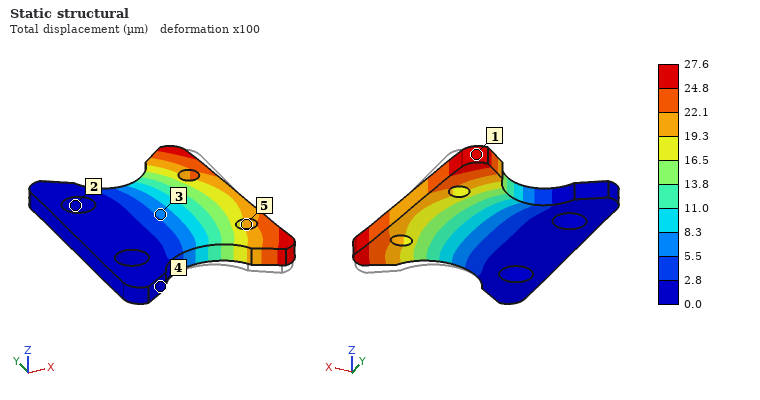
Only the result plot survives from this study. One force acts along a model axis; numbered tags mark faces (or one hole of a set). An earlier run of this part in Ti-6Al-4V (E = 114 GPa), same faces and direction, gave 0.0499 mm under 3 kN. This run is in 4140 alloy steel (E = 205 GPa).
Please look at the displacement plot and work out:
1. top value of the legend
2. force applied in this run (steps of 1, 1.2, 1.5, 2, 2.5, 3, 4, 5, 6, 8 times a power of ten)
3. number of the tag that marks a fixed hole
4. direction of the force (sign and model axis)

27.6 µm
3 kN
2
+Y
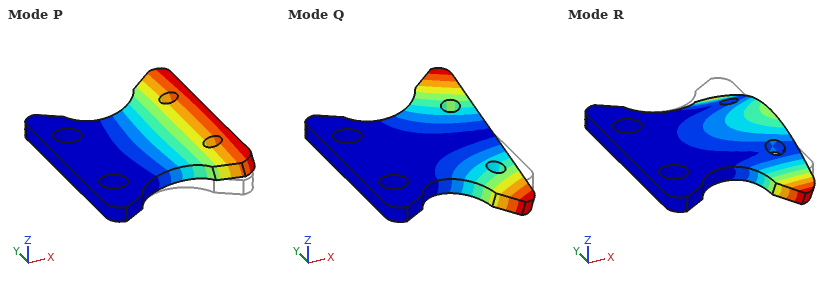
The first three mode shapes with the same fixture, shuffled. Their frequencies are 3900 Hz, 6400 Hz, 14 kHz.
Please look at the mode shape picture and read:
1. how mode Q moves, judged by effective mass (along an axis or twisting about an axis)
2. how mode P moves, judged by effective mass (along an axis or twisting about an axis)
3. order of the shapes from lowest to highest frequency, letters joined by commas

twisting about X
along Z
P, Q, R
